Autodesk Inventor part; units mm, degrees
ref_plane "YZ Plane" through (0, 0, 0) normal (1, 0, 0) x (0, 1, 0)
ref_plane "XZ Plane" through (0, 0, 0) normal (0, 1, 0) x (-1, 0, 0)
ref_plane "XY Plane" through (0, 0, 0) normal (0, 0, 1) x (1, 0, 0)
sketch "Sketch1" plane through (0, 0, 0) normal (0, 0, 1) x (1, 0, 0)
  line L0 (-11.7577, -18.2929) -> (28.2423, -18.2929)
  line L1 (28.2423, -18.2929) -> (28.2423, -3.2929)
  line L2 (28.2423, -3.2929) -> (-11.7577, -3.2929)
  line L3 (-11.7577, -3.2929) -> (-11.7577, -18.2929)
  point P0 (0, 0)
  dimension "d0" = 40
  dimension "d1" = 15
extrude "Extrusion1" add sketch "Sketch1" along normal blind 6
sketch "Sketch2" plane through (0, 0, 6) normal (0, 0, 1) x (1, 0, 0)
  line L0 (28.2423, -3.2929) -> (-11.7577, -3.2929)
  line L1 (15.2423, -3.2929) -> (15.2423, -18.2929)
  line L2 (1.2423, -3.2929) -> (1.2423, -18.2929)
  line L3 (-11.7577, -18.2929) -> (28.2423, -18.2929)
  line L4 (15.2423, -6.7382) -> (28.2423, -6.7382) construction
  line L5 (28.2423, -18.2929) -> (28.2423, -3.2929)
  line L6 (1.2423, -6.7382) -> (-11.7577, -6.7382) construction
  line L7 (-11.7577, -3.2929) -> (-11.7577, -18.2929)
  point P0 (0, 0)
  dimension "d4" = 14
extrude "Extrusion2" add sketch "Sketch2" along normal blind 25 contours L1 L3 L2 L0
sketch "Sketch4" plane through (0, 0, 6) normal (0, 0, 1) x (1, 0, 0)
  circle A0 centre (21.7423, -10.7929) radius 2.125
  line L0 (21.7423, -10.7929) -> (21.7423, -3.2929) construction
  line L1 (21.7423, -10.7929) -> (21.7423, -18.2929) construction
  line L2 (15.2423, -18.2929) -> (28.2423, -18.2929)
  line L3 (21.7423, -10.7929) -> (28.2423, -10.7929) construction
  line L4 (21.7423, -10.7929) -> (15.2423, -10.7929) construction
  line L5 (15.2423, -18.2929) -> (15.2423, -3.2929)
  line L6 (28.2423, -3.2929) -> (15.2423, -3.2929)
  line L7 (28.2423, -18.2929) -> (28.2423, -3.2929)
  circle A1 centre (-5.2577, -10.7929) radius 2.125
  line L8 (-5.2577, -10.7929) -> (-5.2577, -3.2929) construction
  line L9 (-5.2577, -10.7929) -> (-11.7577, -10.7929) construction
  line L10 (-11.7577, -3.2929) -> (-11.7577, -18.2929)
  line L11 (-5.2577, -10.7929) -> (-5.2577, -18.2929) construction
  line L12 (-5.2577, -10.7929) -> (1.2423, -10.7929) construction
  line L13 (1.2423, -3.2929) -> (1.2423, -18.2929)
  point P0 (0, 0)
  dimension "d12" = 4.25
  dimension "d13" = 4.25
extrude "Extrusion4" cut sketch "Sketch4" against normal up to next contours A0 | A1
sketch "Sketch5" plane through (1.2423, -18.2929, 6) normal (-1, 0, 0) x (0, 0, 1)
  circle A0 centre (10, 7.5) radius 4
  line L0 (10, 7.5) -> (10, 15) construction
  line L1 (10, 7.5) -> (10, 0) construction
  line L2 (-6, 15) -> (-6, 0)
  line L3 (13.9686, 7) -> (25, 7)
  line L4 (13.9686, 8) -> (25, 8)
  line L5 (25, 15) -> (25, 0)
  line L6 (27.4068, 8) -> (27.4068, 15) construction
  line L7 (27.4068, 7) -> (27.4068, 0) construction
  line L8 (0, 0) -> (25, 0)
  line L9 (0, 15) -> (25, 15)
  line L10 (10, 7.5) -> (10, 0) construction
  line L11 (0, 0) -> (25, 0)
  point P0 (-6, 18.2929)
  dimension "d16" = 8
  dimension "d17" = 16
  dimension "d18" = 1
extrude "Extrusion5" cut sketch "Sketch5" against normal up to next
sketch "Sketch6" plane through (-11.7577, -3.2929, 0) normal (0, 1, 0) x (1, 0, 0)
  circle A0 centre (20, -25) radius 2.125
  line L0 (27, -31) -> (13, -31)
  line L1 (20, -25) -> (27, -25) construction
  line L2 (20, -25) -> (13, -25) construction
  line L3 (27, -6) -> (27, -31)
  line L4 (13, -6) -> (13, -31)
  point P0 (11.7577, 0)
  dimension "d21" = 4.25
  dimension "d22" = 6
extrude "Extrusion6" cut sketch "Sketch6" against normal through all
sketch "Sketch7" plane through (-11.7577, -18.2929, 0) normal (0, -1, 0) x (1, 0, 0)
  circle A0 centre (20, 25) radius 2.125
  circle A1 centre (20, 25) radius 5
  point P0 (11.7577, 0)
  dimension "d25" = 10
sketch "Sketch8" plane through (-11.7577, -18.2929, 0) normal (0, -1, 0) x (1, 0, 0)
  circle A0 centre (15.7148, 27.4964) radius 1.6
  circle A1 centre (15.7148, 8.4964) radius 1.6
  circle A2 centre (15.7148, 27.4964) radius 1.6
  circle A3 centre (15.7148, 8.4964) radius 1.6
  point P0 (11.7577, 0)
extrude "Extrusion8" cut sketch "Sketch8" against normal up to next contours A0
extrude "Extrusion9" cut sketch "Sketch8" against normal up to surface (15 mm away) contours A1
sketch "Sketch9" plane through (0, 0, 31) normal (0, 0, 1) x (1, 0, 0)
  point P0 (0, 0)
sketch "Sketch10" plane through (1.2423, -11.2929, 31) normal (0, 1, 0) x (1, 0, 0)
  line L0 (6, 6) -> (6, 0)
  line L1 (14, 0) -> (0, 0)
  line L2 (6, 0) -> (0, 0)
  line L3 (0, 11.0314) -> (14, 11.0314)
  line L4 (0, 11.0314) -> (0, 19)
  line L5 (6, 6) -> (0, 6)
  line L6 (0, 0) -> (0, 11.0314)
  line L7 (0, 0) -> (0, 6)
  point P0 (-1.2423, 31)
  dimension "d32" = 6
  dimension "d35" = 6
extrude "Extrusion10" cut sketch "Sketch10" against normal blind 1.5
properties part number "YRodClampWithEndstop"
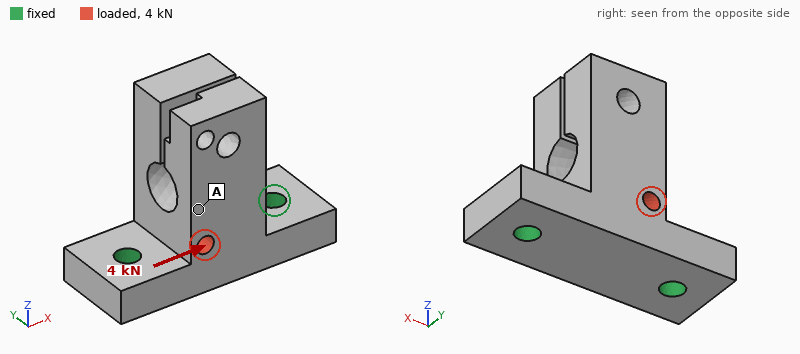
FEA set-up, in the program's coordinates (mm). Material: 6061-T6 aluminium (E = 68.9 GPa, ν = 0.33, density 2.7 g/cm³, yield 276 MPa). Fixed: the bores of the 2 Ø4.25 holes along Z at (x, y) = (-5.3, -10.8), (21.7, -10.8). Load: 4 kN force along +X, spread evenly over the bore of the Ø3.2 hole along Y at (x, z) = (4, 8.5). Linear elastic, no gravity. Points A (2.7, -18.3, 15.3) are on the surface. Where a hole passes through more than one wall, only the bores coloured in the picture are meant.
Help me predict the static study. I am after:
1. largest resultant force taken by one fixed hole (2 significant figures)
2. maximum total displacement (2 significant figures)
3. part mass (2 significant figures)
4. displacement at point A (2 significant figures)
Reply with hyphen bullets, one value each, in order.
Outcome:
- 2.3 kN
- 25 µm
- 20 g
- 14 µm
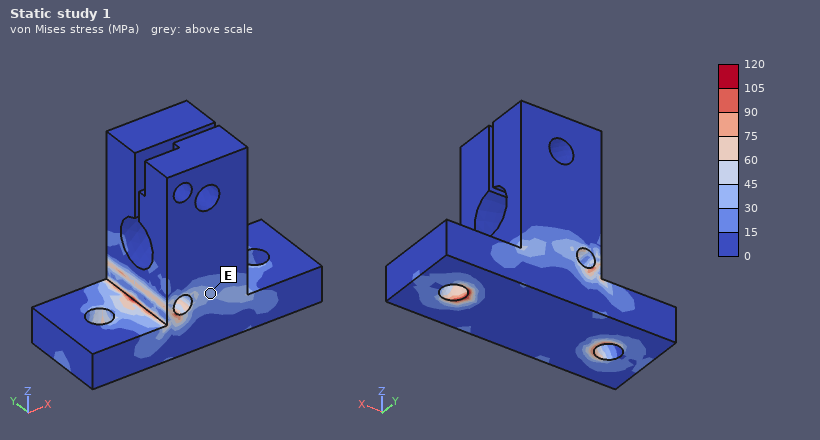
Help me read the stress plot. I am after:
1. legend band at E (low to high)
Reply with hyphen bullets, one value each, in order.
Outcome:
- 30 to 45 MPa
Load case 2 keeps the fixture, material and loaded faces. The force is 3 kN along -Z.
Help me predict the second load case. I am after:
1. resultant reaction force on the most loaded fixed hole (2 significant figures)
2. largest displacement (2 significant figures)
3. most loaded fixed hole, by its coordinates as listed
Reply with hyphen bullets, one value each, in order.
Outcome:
- 2.2 kN
- 27 µm
- (-5.3, -10.8)
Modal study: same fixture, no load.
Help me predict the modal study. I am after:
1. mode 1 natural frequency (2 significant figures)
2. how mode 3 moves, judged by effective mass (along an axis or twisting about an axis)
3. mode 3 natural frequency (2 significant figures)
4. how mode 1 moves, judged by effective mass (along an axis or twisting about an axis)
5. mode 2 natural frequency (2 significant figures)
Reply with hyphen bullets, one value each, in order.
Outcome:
- 4700 Hz
- along X
- 9500 Hz
- along Y
- 6300 Hz
